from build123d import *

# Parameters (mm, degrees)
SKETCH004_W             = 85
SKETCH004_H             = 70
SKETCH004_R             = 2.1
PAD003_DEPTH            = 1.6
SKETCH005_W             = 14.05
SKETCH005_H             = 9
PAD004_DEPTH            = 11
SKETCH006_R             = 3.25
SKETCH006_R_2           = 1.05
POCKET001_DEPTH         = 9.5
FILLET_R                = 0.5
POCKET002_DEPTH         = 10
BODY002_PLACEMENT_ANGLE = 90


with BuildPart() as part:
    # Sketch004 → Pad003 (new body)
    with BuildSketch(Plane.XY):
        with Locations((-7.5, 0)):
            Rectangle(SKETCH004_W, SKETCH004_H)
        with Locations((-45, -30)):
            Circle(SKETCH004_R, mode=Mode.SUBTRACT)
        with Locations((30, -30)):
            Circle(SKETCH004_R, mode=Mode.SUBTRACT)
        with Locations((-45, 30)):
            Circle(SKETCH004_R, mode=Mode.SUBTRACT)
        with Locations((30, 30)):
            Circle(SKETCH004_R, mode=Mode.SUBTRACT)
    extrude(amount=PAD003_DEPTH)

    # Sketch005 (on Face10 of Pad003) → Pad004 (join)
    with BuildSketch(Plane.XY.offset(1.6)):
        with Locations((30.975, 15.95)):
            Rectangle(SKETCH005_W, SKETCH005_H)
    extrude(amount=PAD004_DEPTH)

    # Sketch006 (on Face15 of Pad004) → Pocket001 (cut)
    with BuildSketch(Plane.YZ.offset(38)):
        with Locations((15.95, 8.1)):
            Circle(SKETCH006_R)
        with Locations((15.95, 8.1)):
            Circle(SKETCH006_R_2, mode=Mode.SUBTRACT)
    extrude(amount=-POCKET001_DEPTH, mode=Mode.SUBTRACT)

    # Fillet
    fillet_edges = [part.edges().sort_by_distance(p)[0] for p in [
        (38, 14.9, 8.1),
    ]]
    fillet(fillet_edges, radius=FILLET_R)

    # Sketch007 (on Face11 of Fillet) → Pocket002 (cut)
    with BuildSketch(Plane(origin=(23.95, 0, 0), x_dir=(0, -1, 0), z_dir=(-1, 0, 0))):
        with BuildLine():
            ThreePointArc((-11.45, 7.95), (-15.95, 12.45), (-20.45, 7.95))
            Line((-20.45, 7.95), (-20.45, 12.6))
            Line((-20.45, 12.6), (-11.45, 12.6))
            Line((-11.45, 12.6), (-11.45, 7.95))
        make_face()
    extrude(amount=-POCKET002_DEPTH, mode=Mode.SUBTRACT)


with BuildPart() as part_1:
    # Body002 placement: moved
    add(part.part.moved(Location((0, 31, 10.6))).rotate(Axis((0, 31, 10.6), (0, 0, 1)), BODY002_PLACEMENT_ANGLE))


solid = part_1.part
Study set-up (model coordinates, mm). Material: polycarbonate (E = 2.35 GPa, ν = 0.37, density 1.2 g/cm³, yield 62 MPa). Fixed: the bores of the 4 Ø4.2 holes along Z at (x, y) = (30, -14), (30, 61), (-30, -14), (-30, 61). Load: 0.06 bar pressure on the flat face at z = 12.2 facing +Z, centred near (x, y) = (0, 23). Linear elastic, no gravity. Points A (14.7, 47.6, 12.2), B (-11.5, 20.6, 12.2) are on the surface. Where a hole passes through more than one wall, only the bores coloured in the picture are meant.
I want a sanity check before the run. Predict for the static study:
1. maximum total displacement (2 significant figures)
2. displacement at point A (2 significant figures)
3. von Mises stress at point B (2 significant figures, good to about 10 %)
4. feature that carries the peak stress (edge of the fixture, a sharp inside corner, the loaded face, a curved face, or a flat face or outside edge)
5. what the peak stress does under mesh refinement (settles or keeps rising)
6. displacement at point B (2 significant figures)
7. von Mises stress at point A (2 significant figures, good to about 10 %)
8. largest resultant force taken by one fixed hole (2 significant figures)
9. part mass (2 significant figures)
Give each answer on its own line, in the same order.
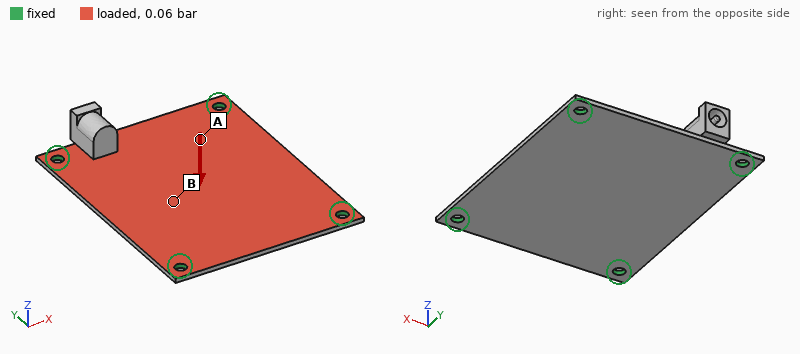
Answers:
0.99 mm
0.50 mm
3.5 MPa
edge of the fixture
keeps rising
0.93 mm
1.5 MPa
8.8 N
13 g
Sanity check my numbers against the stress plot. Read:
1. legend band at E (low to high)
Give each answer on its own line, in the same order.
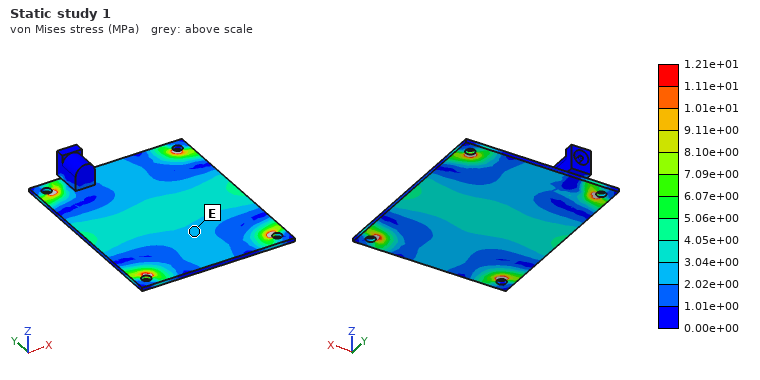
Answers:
2.02e+00 to 3.04e+00 MPa
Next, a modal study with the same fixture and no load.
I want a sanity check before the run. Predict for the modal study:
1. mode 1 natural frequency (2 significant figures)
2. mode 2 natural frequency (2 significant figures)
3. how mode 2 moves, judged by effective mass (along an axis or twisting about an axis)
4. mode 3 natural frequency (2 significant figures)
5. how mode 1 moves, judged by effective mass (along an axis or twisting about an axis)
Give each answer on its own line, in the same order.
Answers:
330 Hz
520 Hz
twisting about Y
600 Hz
along Z
